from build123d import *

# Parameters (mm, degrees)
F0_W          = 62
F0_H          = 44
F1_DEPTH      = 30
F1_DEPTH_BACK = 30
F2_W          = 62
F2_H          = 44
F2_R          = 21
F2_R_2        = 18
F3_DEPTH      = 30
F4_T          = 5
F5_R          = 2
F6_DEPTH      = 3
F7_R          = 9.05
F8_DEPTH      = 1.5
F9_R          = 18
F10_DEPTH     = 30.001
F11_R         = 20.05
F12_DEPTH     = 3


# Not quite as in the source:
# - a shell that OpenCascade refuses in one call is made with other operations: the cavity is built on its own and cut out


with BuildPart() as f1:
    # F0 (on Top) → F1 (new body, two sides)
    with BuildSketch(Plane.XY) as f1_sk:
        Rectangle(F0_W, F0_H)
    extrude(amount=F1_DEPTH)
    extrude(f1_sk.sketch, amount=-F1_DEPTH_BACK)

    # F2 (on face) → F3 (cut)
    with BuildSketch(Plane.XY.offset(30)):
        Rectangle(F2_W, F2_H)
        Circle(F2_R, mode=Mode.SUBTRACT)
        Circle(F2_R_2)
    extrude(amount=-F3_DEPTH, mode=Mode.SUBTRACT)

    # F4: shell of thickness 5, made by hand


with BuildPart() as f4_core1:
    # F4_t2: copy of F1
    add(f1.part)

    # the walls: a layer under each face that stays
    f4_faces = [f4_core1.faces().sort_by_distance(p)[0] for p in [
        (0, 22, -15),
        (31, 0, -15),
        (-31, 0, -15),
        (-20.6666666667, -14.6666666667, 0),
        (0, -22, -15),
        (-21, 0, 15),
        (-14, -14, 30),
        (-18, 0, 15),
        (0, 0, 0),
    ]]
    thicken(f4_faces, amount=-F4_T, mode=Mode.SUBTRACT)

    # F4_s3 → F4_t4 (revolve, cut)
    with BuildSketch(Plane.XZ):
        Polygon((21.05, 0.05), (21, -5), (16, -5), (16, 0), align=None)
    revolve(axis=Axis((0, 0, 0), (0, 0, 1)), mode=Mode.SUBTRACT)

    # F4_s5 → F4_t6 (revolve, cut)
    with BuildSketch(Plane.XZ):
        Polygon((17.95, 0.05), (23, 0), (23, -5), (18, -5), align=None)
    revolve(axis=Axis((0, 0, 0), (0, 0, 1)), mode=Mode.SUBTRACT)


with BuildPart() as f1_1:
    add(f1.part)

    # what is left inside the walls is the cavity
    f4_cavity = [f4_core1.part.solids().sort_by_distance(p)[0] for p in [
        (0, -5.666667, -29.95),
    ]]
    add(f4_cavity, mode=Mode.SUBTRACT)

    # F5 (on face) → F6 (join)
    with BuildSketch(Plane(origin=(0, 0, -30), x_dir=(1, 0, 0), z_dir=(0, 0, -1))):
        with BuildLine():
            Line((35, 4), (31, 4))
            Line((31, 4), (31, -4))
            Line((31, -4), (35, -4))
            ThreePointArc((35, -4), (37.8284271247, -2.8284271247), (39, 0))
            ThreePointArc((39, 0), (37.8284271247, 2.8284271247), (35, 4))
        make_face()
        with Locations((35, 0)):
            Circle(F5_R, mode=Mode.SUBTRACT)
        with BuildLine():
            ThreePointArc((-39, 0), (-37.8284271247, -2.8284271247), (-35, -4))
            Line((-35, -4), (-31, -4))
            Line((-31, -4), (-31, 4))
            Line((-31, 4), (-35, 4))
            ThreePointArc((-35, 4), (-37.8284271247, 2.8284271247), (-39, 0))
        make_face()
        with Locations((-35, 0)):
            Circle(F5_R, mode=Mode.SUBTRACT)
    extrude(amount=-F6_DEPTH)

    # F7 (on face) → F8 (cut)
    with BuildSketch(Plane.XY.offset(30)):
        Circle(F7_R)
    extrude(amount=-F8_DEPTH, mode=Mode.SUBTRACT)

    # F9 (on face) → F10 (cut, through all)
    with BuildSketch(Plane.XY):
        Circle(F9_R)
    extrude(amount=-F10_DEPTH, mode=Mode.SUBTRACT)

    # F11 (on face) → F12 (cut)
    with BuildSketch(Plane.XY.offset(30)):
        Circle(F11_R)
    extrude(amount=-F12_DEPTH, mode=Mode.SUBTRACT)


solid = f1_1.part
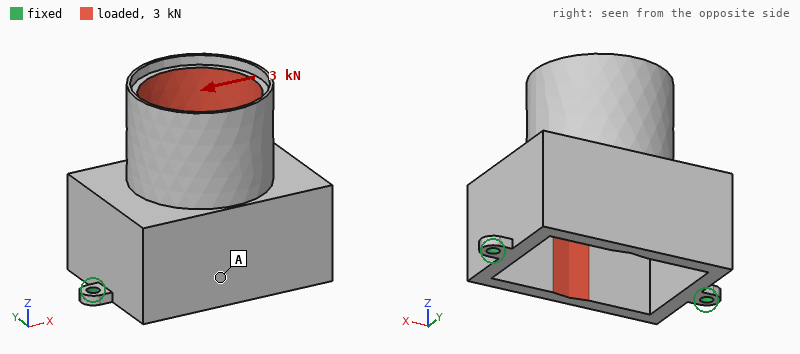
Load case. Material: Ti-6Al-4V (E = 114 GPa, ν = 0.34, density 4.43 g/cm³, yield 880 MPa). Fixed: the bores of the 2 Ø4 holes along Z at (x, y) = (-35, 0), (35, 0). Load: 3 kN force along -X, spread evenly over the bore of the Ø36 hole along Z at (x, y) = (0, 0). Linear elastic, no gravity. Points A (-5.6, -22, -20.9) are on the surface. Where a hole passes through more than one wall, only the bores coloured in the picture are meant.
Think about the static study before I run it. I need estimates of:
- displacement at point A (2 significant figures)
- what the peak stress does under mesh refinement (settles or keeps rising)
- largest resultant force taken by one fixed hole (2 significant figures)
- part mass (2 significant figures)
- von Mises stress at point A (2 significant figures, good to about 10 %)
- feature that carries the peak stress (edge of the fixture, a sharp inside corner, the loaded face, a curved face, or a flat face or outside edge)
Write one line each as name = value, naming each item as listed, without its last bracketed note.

displacement at point A = 35 µm
what the peak stress does under mesh refinement = keeps rising
largest resultant force taken by one fixed hole = 2.2 kN
part mass = 190 g
von Mises stress at point A = 13 MPa
feature that carries the peak stress = edge of the fixture
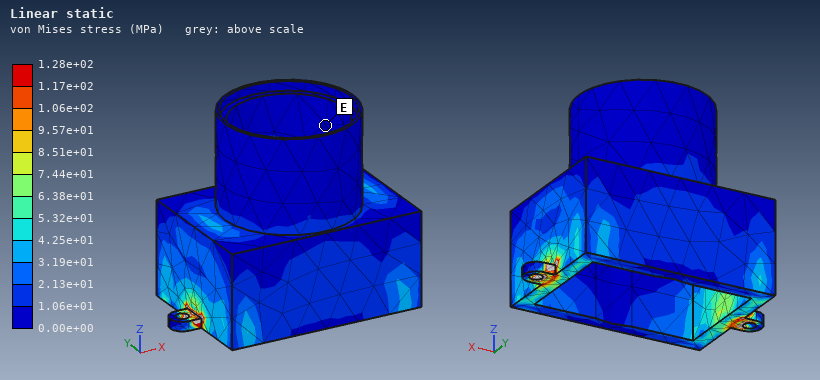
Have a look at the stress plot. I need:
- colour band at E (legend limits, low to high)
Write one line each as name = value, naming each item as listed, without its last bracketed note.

colour band at E = 0.00e+00 to 1.06e+01 MPa
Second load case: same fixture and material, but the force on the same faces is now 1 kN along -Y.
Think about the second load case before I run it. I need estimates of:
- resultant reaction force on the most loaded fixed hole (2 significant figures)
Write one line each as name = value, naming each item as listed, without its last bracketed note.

resultant reaction force on the most loaded fixed hole = 500 N
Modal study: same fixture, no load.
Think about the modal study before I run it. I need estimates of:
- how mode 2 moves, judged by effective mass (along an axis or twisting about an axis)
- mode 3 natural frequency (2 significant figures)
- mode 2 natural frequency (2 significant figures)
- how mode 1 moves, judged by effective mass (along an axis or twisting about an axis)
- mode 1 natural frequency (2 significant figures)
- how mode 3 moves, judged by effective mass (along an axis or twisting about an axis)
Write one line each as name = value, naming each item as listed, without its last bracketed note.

how mode 2 moves, judged by effective mass = along X
mode 3 natural frequency = 3500 Hz
mode 2 natural frequency = 3300 Hz
how mode 1 moves, judged by effective mass = along Y
mode 1 natural frequency = 520 Hz
how mode 3 moves, judged by effective mass = twisting about Z
